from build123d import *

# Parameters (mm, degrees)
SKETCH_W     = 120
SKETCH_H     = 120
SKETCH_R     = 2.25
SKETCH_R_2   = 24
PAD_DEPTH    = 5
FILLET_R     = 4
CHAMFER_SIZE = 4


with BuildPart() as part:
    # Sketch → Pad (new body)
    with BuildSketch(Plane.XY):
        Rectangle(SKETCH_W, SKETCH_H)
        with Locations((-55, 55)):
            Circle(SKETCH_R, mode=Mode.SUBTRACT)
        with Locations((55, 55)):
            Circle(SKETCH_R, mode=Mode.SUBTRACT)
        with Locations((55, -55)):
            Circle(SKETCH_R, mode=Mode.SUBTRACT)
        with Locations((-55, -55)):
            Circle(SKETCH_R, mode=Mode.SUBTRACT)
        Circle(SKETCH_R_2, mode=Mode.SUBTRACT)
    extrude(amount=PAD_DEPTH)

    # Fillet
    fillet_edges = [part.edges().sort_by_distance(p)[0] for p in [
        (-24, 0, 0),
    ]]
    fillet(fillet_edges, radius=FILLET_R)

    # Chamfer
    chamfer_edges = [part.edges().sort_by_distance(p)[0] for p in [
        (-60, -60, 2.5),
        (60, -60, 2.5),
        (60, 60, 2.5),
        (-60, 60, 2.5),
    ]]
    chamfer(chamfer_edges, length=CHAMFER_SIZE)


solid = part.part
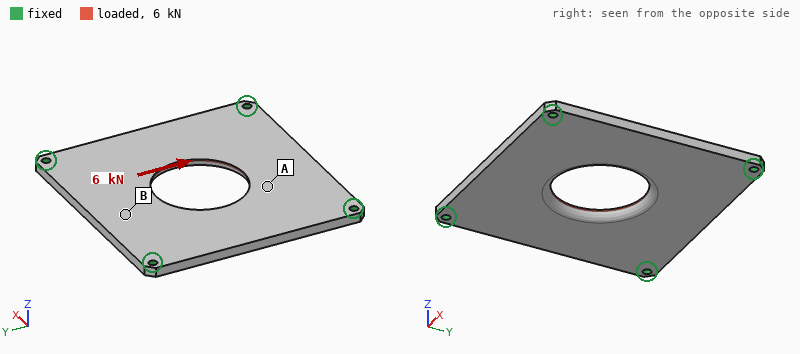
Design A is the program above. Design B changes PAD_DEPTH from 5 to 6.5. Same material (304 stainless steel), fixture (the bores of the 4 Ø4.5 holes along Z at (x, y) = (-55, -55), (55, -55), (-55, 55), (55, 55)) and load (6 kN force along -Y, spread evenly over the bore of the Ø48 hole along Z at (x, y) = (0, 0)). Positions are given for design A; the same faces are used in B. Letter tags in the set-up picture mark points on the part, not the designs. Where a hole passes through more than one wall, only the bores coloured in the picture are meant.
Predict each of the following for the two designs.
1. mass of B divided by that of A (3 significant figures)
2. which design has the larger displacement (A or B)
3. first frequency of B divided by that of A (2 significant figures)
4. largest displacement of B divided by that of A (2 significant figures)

1.30
A
1.3
0.56
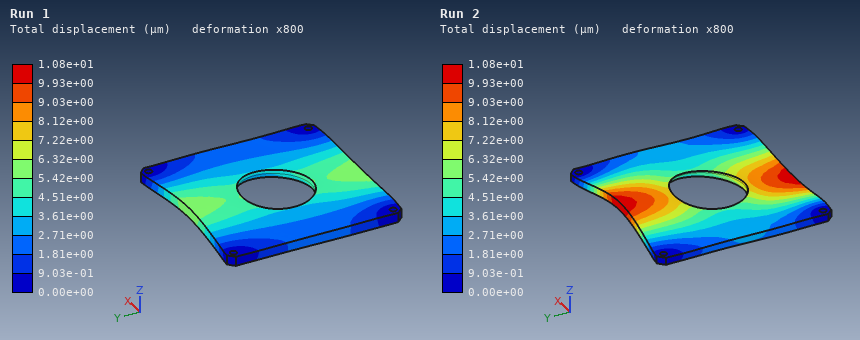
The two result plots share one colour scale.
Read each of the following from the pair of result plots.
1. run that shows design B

Run 1
